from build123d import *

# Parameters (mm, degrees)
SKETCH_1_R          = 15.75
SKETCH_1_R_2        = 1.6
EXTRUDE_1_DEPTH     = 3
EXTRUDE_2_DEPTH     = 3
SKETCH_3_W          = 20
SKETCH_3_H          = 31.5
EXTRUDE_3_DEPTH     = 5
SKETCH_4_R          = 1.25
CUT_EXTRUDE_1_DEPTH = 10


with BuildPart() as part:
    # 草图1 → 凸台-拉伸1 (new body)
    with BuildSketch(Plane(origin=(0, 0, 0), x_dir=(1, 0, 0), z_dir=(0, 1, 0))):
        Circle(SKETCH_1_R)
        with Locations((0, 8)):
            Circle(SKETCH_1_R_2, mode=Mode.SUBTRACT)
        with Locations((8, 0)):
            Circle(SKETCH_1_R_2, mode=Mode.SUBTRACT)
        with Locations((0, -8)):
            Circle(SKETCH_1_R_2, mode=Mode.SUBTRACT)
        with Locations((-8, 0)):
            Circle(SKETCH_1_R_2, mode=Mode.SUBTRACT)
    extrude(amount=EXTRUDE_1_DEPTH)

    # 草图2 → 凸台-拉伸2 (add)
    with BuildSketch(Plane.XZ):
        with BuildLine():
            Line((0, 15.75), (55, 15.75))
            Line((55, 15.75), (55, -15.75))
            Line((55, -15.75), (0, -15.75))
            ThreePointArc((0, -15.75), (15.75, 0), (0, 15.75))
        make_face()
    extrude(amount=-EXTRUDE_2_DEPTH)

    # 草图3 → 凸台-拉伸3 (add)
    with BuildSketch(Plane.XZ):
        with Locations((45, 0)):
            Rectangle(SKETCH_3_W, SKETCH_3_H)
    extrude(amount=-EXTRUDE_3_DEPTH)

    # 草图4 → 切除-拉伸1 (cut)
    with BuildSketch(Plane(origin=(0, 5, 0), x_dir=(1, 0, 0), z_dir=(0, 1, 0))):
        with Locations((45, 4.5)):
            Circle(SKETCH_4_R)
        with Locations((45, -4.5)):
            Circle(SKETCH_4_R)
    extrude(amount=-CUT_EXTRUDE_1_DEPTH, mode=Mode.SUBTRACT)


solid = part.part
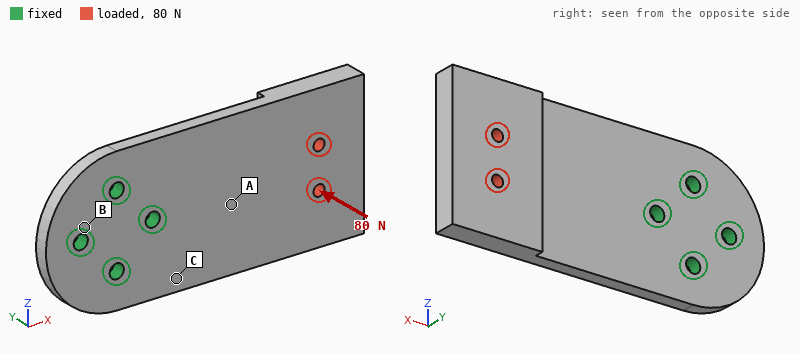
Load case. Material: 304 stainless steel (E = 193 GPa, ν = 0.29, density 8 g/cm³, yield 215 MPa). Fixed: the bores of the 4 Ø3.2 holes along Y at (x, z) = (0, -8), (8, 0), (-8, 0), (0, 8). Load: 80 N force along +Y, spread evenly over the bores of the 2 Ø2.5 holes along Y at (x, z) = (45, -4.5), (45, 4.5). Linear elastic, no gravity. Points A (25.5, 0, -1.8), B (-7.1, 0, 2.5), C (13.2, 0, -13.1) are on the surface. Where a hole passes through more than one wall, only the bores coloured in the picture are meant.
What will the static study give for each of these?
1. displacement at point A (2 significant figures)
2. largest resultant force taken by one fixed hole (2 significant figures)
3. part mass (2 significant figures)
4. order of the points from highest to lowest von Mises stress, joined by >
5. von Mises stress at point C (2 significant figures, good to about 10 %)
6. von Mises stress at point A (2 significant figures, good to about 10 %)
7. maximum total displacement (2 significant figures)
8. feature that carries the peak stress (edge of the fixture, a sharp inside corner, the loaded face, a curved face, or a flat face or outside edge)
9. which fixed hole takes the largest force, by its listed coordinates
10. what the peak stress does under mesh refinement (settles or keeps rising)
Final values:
0.032 mm
240 N
60 g
C > A > B
44 MPa
28 MPa
0.14 mm
edge of the fixture
(8, 0)
keeps rising
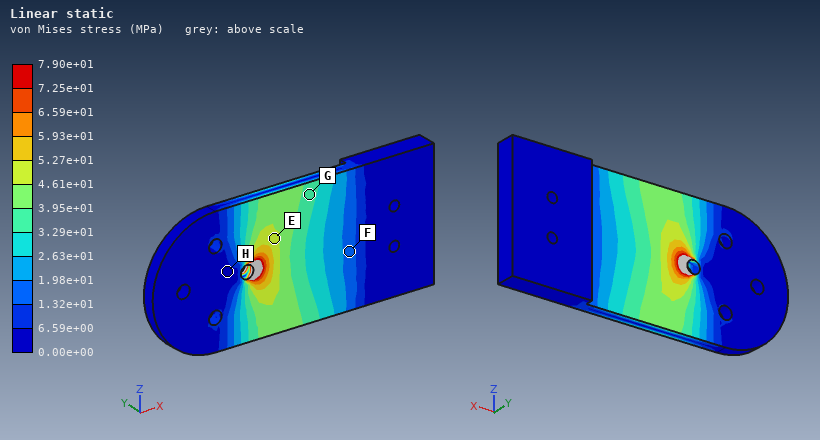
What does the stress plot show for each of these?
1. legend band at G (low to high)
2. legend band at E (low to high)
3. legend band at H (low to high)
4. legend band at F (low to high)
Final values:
3.29e+01 to 3.95e+01 MPa
4.61e+01 to 5.27e+01 MPa
0.00e+00 to 6.59e+00 MPa
1.32e+01 to 1.98e+01 MPa
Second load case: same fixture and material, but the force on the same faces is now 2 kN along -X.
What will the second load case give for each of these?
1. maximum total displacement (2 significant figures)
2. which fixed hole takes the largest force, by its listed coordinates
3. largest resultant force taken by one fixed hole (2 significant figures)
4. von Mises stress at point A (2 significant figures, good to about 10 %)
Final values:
0.14 mm
(8, 0)
910 N
16 MPa
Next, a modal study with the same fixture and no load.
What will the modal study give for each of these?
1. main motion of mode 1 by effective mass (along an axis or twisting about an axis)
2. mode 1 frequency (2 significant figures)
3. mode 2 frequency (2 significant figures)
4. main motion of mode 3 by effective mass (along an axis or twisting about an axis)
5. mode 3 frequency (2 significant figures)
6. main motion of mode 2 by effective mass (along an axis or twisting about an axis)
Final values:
along Y
840 Hz
2700 Hz
along Z
5500 Hz
twisting about X
